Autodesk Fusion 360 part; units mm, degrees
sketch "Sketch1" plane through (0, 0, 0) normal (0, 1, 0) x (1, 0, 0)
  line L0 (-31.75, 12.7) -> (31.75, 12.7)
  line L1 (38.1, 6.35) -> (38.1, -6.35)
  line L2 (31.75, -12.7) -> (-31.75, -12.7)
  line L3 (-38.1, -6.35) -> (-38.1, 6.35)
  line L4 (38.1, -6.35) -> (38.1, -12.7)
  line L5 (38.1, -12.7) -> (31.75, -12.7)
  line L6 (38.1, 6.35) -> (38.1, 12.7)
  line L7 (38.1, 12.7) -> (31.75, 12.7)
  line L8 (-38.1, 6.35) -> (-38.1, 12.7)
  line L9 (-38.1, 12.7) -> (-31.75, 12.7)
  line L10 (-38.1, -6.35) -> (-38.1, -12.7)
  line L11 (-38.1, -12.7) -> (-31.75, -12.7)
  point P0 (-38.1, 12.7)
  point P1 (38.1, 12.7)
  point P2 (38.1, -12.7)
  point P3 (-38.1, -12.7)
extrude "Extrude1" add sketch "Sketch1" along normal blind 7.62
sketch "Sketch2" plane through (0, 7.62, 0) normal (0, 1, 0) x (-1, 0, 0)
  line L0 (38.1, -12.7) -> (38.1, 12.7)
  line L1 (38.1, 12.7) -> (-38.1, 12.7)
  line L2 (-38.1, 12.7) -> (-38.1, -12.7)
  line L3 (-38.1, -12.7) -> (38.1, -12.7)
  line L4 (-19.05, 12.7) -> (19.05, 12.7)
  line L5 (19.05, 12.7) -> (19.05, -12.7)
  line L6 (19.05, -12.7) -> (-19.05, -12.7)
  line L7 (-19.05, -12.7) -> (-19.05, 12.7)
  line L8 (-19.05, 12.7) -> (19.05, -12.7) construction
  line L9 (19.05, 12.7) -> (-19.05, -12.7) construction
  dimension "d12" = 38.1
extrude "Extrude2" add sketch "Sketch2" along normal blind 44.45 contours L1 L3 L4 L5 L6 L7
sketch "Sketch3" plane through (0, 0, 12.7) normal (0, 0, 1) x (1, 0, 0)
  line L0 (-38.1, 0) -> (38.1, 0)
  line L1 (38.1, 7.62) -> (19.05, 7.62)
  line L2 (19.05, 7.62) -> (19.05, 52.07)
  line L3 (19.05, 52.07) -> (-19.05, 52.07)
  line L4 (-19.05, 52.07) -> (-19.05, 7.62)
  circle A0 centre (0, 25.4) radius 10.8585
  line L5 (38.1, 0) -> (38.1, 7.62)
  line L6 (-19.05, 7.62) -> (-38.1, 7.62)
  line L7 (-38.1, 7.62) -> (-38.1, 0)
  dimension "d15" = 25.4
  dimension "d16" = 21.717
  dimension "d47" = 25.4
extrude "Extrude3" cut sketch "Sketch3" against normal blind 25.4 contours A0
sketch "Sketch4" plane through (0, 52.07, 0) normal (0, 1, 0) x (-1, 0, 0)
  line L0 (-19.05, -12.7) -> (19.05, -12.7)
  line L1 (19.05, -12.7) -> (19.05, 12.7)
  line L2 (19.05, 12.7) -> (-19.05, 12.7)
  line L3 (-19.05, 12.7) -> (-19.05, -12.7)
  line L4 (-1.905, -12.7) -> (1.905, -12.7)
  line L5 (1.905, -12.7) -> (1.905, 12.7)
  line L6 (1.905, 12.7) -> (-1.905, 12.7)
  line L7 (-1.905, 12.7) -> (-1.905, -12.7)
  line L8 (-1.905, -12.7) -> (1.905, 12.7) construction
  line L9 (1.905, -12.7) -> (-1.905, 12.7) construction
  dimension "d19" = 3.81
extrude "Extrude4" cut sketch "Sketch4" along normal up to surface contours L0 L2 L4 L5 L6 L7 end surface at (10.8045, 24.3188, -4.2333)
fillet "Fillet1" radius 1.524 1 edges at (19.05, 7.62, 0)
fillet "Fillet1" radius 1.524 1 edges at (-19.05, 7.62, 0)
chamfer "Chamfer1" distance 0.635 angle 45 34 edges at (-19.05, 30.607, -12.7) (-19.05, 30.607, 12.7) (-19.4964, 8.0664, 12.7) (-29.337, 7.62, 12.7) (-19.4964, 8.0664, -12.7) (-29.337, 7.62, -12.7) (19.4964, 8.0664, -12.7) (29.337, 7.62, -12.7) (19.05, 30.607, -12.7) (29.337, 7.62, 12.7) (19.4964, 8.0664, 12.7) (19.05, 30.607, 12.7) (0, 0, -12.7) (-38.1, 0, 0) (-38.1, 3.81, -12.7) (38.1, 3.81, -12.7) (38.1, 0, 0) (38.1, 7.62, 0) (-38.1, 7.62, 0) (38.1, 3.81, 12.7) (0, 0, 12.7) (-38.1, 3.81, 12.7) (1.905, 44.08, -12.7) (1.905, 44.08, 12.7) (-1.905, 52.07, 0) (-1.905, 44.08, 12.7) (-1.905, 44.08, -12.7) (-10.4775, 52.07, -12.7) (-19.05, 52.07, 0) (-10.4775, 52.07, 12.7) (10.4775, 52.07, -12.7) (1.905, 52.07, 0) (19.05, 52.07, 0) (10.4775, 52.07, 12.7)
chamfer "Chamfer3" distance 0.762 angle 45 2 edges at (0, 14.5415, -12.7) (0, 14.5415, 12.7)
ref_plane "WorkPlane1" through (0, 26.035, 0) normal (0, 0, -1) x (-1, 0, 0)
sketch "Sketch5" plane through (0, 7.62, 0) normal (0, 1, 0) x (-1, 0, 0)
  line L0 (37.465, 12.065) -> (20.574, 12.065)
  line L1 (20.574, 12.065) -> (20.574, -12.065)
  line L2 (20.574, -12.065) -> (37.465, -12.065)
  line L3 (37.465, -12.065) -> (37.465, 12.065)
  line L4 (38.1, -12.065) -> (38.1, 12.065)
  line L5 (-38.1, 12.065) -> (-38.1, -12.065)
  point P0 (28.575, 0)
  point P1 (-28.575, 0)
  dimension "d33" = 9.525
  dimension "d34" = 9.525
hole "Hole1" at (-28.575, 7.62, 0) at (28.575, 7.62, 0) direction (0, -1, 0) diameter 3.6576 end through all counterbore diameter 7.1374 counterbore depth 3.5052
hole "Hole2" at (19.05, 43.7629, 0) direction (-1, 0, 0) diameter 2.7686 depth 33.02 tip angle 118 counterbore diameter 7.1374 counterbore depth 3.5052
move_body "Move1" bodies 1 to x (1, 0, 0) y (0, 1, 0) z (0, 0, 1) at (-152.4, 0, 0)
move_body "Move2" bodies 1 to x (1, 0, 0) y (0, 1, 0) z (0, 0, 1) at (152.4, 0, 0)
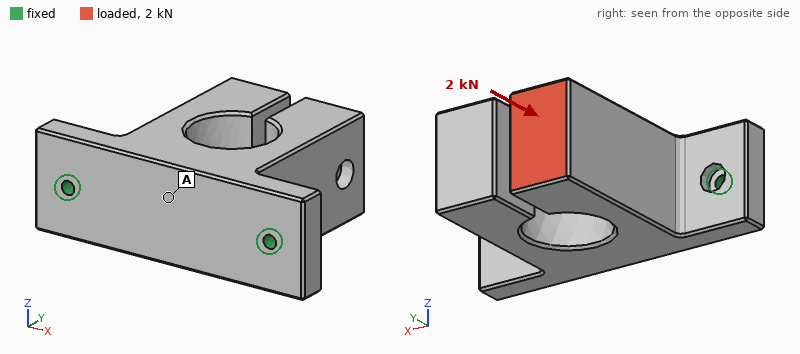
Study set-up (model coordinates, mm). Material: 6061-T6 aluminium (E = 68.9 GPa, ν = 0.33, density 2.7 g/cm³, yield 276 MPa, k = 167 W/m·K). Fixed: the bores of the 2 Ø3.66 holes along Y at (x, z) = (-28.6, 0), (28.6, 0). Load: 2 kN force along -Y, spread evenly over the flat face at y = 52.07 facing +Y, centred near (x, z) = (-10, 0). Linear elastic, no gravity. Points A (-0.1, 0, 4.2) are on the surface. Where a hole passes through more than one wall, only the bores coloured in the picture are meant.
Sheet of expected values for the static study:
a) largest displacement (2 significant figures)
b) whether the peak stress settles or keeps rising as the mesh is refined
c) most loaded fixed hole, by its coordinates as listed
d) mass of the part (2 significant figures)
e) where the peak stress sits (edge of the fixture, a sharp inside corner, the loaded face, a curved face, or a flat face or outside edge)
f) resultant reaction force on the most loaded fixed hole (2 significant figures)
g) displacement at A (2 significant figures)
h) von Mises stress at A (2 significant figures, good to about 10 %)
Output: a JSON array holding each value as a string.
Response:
["57 µm", "keeps rising", "(-28.6, 0)", "120 g", "edge of the fixture", "1.7 kN", "14 µm", "8.4 MPa"]
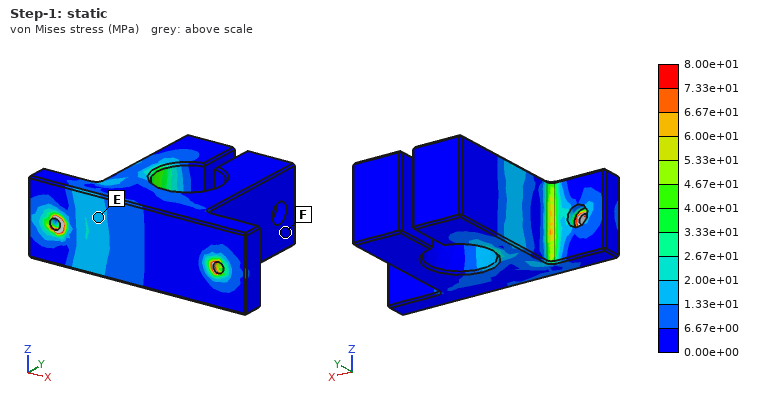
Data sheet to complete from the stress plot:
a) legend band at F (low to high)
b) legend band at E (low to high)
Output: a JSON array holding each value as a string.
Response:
["0.00e+00 to 6.67e+00 MPa", "1.33e+01 to 2.00e+01 MPa"]
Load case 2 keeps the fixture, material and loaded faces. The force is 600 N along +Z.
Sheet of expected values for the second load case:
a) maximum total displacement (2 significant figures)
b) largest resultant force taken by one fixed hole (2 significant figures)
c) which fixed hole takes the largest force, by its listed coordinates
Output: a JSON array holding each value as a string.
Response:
["0.30 mm", "400 N", "(-28.6, 0)"]
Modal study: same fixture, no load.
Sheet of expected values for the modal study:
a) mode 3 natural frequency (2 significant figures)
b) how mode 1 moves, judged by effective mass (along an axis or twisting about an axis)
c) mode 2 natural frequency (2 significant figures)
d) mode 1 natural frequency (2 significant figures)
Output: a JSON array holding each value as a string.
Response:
["3200 Hz", "along Z", "3200 Hz", "1300 Hz"]
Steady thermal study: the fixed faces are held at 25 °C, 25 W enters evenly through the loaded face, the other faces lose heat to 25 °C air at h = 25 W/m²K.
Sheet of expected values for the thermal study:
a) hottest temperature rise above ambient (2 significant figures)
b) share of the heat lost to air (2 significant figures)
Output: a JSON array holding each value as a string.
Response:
["30 K", "12 %"]
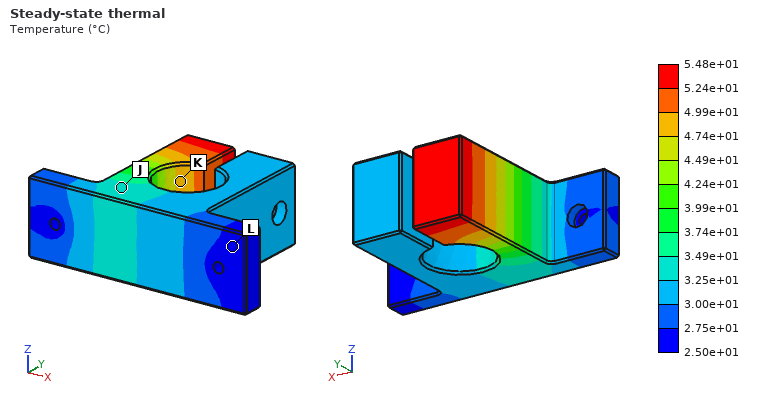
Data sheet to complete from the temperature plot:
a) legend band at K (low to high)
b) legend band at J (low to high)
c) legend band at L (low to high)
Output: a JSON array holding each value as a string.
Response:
["4.74e+01 to 4.99e+01 °C", "3.25e+01 to 3.49e+01 °C", "2.50e+01 to 2.75e+01 °C"]
